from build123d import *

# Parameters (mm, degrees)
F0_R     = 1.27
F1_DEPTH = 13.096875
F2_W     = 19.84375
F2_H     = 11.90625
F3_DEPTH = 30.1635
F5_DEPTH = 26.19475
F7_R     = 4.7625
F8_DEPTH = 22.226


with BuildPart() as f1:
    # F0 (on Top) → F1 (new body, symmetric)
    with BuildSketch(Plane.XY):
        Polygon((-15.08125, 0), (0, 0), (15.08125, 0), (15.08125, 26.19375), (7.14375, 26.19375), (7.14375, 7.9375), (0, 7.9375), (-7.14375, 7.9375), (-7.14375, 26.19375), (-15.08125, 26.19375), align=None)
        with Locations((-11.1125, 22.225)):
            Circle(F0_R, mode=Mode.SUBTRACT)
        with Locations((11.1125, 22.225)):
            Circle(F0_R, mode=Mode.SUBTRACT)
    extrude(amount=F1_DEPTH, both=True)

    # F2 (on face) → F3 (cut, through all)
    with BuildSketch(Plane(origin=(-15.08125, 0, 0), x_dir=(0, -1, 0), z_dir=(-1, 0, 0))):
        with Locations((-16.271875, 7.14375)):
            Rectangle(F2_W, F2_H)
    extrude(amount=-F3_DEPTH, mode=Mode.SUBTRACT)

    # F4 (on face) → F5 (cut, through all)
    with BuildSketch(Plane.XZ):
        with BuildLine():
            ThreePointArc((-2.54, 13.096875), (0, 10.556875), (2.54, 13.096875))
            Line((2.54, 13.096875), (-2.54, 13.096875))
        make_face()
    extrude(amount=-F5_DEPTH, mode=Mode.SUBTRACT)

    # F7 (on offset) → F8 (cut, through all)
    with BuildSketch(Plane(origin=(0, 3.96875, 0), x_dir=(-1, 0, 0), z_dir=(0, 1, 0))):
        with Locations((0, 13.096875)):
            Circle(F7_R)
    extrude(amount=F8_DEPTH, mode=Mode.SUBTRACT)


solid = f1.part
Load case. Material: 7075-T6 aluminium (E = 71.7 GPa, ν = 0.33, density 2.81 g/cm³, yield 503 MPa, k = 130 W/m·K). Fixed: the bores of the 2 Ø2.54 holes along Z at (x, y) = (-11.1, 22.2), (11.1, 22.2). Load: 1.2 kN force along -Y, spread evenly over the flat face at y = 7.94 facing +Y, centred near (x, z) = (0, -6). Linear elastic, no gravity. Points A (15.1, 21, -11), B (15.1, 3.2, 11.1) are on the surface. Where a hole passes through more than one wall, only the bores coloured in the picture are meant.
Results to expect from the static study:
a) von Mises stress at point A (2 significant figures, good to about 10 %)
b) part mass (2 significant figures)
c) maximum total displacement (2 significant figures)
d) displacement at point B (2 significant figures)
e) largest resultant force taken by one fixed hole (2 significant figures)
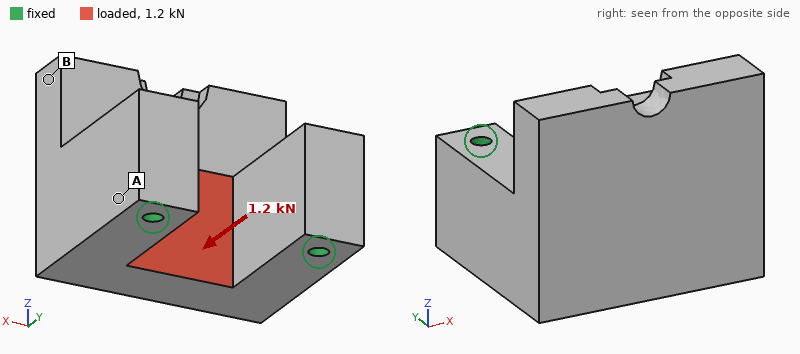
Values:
3.9 MPa
27 g
4.5 µm
1.0 µm
620 N
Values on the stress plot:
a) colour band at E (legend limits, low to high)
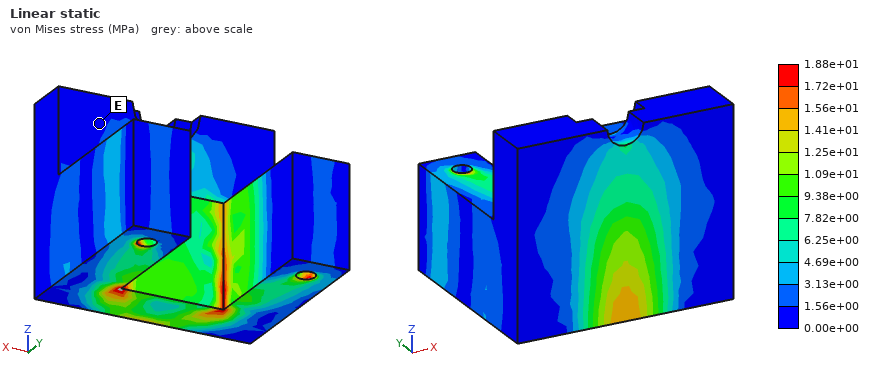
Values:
0.00e+00 to 1.56e+00 MPa
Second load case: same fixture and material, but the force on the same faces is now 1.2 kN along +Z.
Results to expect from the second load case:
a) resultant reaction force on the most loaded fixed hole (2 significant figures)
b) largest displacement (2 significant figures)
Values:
600 N
14 µm
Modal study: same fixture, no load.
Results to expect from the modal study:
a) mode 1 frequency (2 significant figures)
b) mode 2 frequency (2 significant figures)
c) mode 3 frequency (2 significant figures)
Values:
9600 Hz
9800 Hz
15 kHz
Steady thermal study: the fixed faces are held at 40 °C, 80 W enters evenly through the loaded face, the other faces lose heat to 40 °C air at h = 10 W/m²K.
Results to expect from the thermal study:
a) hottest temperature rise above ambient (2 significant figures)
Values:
64 K
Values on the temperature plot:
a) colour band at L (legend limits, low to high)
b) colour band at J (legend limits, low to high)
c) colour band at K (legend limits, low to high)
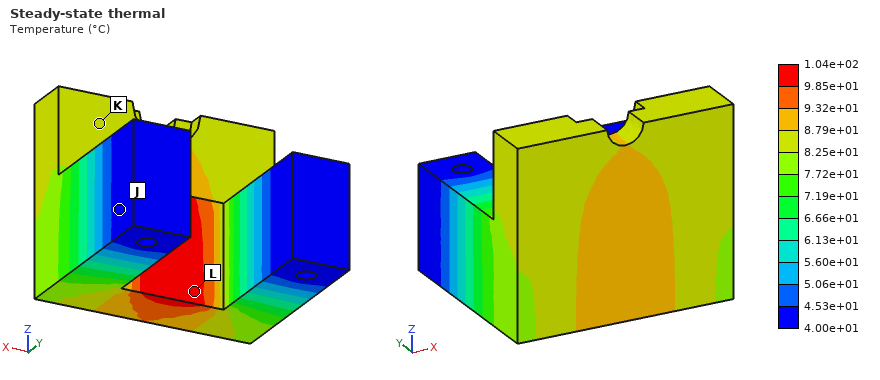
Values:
9.85e+01 to 1.04e+02 °C
4.00e+01 to 4.53e+01 °C
8.25e+01 to 8.79e+01 °C
